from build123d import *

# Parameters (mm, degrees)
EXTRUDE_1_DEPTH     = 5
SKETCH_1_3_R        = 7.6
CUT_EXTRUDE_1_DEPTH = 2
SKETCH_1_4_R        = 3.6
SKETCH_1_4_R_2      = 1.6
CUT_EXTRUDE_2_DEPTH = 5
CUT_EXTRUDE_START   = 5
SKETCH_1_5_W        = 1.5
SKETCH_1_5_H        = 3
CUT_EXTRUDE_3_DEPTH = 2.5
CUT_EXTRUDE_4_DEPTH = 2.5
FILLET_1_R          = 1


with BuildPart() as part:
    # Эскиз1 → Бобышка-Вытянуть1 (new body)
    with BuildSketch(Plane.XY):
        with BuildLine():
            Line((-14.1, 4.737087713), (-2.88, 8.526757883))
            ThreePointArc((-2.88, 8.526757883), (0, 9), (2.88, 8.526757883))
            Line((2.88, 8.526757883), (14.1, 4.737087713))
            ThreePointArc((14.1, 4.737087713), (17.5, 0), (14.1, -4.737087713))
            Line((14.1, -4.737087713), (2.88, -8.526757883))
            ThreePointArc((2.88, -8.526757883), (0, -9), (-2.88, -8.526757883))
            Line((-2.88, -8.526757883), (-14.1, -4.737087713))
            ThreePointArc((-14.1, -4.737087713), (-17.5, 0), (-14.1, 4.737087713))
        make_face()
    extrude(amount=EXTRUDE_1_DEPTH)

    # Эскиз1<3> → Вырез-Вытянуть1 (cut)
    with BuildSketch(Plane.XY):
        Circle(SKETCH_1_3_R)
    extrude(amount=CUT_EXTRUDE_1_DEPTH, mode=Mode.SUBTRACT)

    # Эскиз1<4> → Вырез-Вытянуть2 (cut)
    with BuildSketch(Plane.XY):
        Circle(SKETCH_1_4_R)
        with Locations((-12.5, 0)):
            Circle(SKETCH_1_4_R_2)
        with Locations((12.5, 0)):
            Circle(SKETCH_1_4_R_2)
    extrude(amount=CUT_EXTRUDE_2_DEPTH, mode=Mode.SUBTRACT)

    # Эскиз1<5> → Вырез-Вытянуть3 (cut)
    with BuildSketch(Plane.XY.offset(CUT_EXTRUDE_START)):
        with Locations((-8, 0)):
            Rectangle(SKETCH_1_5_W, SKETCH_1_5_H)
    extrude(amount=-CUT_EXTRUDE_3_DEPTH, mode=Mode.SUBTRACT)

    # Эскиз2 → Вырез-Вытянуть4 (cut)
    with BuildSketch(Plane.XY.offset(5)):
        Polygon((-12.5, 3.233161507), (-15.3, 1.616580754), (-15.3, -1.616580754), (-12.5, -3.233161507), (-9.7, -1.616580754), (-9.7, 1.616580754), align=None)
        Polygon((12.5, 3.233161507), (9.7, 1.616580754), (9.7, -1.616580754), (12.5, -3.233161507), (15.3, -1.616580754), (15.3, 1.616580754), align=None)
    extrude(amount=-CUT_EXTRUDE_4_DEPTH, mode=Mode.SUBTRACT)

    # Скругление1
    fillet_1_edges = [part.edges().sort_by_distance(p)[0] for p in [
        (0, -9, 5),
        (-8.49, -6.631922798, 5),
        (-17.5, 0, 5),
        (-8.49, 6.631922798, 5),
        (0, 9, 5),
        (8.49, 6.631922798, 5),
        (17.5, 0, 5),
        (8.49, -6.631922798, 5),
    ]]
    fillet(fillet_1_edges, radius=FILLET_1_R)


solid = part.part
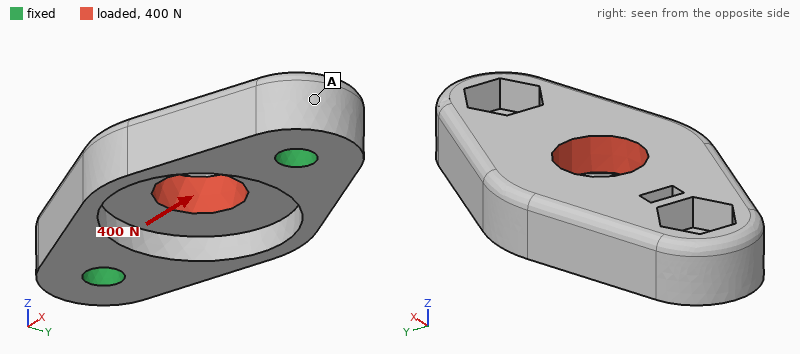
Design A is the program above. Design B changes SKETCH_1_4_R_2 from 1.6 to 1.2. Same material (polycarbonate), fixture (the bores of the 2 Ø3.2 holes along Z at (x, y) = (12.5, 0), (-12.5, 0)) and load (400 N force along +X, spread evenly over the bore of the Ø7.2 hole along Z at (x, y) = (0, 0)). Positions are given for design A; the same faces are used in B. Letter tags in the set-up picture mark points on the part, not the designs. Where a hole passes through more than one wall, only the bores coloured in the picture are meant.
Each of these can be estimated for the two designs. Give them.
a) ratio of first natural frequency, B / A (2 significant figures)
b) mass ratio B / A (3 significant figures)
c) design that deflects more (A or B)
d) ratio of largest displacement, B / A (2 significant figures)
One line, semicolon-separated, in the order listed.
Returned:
0.88; 1.01; B; 1.1
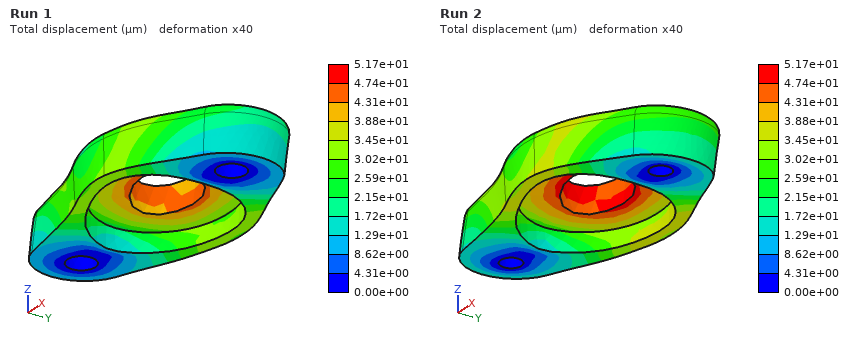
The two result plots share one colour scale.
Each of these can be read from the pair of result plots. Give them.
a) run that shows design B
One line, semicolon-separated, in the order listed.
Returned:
Run 2
